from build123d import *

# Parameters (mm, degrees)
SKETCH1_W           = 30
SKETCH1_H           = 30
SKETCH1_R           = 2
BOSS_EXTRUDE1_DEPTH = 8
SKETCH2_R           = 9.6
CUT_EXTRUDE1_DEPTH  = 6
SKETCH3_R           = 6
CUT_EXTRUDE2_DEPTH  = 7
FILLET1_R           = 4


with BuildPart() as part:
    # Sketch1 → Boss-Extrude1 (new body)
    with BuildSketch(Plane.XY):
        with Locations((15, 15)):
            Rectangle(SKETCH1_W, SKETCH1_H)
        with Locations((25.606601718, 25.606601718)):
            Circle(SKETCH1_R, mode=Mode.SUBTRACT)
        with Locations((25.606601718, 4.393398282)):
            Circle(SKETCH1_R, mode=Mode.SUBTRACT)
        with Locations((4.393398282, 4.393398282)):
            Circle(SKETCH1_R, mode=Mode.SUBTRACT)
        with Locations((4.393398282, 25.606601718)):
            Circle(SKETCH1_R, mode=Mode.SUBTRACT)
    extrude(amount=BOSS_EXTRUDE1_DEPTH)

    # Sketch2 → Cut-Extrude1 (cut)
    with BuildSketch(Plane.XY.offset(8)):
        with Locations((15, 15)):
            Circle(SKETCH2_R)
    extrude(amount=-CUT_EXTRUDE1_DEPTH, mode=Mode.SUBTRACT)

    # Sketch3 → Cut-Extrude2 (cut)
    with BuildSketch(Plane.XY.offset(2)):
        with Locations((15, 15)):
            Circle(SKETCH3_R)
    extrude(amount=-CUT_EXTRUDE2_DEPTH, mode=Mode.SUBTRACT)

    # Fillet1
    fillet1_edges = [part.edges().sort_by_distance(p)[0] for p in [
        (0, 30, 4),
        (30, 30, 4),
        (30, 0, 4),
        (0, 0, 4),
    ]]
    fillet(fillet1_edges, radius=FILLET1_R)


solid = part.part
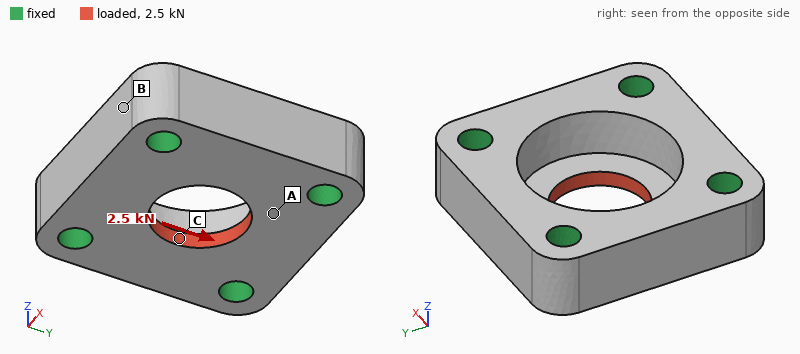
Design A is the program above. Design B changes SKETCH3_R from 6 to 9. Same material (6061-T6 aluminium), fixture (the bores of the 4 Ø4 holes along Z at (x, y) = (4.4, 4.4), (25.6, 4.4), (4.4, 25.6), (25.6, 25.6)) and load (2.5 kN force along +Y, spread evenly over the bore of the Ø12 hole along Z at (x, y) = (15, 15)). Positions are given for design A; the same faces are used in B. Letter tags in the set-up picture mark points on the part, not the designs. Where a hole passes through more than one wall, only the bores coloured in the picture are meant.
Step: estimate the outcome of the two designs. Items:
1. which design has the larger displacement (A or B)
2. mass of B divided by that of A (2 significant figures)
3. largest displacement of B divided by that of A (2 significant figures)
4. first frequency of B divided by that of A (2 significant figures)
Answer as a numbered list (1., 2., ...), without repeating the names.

1. A
2. 0.94
3. 0.81
4. 0.99
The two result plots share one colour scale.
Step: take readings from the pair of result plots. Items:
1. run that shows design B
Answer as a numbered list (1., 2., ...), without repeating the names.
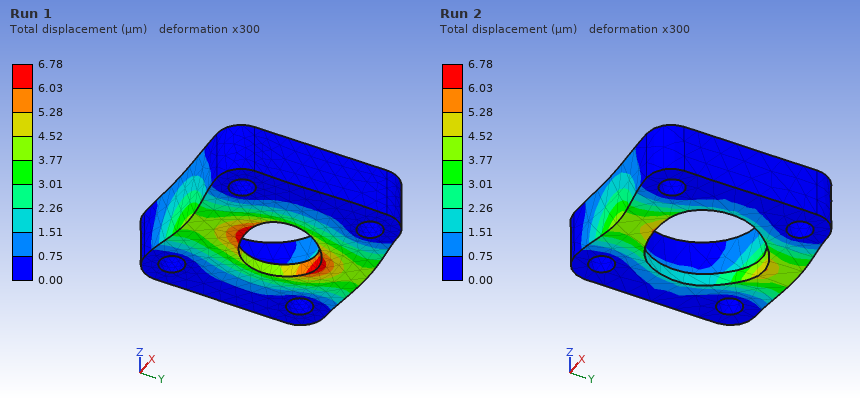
1. Run 2
